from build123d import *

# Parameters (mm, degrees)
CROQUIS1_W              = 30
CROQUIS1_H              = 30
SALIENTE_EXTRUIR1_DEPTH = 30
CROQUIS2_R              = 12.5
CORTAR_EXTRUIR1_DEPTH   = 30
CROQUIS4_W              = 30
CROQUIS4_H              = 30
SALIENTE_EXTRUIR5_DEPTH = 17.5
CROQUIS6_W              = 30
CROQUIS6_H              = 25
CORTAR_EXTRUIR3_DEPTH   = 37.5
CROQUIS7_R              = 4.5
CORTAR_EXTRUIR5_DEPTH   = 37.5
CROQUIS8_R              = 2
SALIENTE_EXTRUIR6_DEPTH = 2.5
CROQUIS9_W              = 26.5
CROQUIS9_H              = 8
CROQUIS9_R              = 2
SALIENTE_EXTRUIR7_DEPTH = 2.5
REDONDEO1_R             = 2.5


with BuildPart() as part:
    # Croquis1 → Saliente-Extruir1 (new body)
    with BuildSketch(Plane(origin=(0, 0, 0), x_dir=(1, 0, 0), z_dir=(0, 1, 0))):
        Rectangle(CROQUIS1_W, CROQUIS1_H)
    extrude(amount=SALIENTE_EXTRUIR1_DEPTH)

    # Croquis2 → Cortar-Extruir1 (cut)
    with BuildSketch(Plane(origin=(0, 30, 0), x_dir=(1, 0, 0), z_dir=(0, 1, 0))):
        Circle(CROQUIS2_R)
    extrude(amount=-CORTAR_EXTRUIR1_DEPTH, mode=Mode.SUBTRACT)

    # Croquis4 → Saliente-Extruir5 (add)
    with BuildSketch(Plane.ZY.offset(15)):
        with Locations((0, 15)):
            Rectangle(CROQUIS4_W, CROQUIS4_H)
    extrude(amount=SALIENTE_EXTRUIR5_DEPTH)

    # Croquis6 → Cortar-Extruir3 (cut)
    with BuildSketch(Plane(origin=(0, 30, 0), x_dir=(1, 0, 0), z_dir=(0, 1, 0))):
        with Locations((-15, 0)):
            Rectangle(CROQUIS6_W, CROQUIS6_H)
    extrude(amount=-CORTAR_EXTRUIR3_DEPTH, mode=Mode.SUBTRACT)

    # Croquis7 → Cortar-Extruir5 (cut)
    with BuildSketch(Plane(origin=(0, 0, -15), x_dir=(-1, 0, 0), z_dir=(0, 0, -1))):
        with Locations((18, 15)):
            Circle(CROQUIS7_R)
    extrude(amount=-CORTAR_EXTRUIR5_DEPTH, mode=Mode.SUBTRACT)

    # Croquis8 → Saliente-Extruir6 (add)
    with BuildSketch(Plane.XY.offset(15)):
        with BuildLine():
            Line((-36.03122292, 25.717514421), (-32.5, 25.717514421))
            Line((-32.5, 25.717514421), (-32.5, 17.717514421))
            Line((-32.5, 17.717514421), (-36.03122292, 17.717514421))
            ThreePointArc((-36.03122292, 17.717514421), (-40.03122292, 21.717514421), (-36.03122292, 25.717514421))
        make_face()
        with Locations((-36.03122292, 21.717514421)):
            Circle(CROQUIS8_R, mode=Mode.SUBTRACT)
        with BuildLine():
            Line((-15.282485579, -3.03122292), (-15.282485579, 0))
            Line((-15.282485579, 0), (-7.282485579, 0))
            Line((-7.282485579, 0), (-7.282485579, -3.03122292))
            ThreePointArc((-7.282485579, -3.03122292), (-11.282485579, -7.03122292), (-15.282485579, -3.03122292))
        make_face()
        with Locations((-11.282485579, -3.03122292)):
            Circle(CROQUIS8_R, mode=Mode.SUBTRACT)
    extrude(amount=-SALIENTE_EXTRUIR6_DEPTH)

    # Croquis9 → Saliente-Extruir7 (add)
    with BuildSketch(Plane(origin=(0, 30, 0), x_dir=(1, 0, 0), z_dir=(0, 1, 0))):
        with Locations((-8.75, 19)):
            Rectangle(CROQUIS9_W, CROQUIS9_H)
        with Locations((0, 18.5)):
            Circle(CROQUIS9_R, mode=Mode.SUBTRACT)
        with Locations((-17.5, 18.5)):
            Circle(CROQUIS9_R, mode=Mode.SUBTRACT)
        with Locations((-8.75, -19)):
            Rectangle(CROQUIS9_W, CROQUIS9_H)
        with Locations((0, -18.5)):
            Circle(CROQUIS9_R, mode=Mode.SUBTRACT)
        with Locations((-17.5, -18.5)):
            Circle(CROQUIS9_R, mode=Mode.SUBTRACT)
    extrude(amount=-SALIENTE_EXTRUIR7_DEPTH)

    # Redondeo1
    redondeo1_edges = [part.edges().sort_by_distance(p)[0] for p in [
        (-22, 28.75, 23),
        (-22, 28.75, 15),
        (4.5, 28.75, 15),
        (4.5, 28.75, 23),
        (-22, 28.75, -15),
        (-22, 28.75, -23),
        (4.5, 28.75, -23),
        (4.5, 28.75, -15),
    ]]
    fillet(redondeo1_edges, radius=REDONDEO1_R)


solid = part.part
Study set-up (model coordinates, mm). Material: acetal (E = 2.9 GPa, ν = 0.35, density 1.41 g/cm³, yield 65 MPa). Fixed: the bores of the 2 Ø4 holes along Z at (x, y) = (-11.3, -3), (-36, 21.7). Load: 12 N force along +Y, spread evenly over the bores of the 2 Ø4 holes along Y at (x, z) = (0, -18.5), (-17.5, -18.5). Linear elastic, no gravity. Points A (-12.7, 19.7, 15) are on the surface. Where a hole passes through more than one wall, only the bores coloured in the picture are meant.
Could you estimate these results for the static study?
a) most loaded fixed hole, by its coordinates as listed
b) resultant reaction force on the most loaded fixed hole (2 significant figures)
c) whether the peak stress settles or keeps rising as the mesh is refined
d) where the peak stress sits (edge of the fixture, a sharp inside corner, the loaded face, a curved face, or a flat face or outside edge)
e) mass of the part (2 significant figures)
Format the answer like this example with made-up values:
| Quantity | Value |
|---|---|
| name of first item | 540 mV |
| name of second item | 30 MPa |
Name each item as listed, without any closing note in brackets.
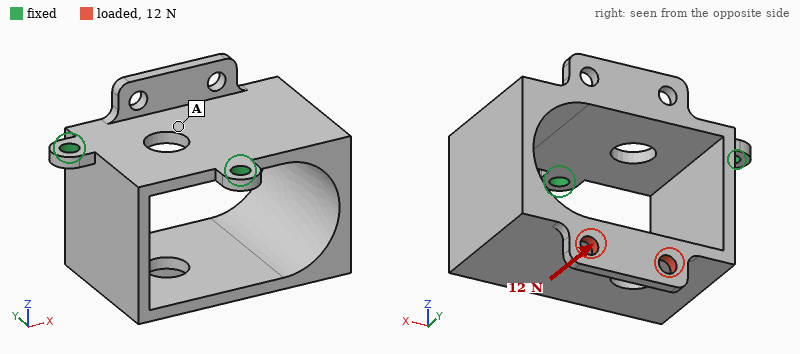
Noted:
| Quantity | Value |
|---|---|
| most loaded fixed hole, by its coordinates as listed | (-11.3, -3) |
| resultant reaction force on the most loaded fixed hole | 10 N |
| whether the peak stress settles or keeps rising as the mesh is refined | keeps rising |
| where the peak stress sits | edge of the fixture |
| mass of the part | 19 g |
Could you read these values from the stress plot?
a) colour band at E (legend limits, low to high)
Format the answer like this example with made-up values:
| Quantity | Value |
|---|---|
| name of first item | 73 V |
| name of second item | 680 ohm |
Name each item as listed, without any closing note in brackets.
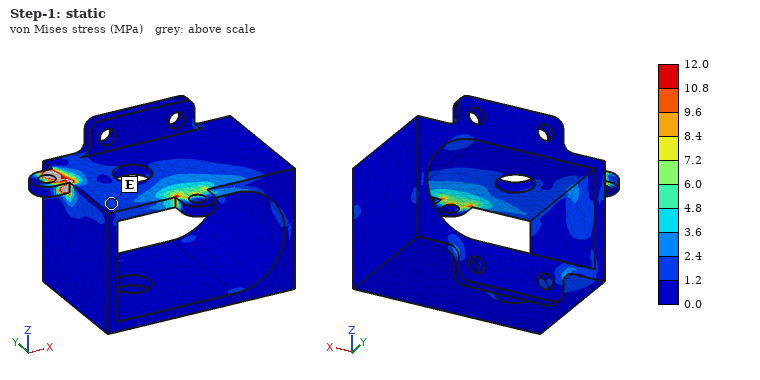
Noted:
| Quantity | Value |
|---|---|
| colour band at E | 1.2 to 2.4 MPa |
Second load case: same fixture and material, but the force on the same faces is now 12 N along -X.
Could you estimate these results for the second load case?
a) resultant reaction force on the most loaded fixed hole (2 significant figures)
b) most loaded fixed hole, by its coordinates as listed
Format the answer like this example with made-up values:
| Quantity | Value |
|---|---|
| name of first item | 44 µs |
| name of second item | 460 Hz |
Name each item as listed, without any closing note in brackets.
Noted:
| Quantity | Value |
|---|---|
| resultant reaction force on the most loaded fixed hole | 17 N |
| most loaded fixed hole, by its coordinates as listed | (-36, 21.7) |
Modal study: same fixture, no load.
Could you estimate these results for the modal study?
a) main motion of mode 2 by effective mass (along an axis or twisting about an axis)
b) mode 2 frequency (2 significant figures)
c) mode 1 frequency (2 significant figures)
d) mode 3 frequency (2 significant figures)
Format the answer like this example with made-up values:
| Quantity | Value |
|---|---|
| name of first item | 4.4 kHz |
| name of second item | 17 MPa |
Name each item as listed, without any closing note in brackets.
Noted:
| Quantity | Value |
|---|---|
| main motion of mode 2 by effective mass | along Y |
| mode 2 frequency | 410 Hz |
| mode 1 frequency | 170 Hz |
| mode 3 frequency | 750 Hz |
